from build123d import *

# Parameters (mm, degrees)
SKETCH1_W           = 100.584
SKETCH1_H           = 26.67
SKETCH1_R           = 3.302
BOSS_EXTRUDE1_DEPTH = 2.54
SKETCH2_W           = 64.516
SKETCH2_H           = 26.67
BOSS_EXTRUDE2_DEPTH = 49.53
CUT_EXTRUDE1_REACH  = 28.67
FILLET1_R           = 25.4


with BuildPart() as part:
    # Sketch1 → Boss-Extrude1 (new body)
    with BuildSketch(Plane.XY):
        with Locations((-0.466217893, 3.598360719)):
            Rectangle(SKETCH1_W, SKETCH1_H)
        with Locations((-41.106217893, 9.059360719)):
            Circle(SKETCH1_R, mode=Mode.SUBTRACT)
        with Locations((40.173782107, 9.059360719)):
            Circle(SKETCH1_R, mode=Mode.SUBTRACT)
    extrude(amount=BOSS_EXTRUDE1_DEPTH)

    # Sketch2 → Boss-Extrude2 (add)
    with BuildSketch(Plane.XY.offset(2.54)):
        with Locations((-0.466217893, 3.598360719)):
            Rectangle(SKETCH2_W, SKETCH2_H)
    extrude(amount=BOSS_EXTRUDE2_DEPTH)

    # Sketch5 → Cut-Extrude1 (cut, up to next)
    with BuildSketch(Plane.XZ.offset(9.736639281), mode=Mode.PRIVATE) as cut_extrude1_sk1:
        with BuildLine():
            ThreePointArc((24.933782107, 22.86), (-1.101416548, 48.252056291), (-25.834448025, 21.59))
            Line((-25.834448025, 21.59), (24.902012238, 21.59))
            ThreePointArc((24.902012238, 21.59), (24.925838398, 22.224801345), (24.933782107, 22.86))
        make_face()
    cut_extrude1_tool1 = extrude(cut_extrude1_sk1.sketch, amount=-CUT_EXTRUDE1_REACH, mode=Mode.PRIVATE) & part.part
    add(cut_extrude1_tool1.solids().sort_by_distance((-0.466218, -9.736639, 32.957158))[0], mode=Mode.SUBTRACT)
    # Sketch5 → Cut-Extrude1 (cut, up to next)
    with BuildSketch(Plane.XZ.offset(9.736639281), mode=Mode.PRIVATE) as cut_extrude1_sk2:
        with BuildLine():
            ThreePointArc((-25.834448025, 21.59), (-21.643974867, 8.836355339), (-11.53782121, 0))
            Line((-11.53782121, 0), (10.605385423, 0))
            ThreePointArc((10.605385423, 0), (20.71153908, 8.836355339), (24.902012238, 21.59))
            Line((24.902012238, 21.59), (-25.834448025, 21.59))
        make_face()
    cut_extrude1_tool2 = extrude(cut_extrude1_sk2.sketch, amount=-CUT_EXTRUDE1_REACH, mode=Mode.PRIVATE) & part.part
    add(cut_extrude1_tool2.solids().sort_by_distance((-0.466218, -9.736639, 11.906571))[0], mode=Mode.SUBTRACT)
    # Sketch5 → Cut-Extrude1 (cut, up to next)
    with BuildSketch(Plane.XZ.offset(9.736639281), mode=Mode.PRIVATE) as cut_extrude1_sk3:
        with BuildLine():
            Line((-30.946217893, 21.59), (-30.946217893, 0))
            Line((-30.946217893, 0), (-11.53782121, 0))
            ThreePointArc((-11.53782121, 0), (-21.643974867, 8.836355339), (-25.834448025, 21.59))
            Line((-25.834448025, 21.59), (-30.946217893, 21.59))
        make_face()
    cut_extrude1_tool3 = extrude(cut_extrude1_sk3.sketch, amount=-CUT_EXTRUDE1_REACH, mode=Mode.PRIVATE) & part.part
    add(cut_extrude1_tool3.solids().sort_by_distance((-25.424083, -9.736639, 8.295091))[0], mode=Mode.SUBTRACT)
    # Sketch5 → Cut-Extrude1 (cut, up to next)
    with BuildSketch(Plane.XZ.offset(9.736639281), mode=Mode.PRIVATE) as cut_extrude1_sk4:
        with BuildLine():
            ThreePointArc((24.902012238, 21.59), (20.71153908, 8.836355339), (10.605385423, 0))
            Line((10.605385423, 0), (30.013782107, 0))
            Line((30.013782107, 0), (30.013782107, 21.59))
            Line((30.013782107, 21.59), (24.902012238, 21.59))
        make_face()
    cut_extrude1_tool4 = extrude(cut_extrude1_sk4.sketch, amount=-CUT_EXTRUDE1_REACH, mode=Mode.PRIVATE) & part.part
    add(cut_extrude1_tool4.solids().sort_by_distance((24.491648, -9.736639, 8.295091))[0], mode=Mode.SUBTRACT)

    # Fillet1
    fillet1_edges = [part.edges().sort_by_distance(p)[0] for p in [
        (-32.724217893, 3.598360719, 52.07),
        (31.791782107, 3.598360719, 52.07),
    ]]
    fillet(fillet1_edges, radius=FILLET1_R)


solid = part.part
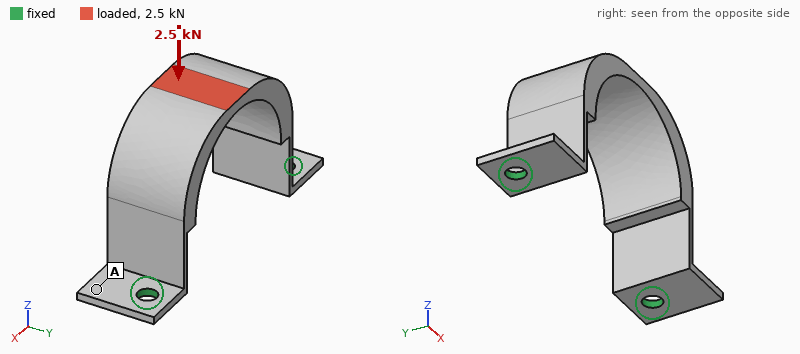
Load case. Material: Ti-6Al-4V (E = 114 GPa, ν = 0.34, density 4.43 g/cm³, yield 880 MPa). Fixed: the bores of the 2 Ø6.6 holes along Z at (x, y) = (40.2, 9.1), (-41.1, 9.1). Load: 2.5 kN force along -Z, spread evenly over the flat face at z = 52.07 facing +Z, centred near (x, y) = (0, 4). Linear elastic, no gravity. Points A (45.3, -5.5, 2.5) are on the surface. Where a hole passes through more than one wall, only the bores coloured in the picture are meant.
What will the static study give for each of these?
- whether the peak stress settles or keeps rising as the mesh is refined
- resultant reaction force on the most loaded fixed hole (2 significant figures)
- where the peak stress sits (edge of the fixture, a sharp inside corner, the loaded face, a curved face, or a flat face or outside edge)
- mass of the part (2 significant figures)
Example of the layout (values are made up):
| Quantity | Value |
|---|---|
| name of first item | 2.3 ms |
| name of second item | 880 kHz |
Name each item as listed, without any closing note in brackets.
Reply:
| Quantity | Value |
|---|---|
| whether the peak stress settles or keeps rising as the mesh is refined | keeps rising |
| resultant reaction force on the most loaded fixed hole | 1.4 kN |
| where the peak stress sits | edge of the fixture |
| mass of the part | 91 g |
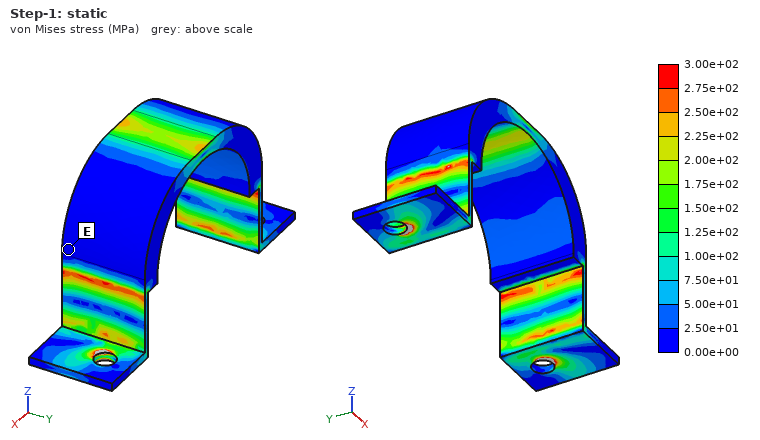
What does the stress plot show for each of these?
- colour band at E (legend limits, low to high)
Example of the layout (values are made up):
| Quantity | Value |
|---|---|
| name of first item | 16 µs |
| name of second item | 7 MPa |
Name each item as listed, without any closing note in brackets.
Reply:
| Quantity | Value |
|---|---|
| colour band at E | 0.00e+00 to 2.50e+01 MPa |
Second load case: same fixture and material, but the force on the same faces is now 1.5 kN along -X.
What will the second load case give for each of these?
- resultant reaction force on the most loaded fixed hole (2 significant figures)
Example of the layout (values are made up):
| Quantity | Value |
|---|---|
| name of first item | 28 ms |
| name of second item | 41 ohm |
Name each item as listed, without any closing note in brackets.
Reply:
| Quantity | Value |
|---|---|
| resultant reaction force on the most loaded fixed hole | 1.2 kN |
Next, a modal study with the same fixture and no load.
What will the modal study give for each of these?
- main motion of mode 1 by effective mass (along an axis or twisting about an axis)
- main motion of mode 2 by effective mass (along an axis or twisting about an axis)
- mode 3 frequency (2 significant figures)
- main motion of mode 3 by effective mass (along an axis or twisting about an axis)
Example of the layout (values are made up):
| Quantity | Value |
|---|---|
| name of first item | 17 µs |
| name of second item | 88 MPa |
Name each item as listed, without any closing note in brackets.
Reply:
| Quantity | Value |
|---|---|
| main motion of mode 1 by effective mass | along Y |
| main motion of mode 2 by effective mass | along X |
| mode 3 frequency | 1900 Hz |
| main motion of mode 3 by effective mass | twisting about Z |
